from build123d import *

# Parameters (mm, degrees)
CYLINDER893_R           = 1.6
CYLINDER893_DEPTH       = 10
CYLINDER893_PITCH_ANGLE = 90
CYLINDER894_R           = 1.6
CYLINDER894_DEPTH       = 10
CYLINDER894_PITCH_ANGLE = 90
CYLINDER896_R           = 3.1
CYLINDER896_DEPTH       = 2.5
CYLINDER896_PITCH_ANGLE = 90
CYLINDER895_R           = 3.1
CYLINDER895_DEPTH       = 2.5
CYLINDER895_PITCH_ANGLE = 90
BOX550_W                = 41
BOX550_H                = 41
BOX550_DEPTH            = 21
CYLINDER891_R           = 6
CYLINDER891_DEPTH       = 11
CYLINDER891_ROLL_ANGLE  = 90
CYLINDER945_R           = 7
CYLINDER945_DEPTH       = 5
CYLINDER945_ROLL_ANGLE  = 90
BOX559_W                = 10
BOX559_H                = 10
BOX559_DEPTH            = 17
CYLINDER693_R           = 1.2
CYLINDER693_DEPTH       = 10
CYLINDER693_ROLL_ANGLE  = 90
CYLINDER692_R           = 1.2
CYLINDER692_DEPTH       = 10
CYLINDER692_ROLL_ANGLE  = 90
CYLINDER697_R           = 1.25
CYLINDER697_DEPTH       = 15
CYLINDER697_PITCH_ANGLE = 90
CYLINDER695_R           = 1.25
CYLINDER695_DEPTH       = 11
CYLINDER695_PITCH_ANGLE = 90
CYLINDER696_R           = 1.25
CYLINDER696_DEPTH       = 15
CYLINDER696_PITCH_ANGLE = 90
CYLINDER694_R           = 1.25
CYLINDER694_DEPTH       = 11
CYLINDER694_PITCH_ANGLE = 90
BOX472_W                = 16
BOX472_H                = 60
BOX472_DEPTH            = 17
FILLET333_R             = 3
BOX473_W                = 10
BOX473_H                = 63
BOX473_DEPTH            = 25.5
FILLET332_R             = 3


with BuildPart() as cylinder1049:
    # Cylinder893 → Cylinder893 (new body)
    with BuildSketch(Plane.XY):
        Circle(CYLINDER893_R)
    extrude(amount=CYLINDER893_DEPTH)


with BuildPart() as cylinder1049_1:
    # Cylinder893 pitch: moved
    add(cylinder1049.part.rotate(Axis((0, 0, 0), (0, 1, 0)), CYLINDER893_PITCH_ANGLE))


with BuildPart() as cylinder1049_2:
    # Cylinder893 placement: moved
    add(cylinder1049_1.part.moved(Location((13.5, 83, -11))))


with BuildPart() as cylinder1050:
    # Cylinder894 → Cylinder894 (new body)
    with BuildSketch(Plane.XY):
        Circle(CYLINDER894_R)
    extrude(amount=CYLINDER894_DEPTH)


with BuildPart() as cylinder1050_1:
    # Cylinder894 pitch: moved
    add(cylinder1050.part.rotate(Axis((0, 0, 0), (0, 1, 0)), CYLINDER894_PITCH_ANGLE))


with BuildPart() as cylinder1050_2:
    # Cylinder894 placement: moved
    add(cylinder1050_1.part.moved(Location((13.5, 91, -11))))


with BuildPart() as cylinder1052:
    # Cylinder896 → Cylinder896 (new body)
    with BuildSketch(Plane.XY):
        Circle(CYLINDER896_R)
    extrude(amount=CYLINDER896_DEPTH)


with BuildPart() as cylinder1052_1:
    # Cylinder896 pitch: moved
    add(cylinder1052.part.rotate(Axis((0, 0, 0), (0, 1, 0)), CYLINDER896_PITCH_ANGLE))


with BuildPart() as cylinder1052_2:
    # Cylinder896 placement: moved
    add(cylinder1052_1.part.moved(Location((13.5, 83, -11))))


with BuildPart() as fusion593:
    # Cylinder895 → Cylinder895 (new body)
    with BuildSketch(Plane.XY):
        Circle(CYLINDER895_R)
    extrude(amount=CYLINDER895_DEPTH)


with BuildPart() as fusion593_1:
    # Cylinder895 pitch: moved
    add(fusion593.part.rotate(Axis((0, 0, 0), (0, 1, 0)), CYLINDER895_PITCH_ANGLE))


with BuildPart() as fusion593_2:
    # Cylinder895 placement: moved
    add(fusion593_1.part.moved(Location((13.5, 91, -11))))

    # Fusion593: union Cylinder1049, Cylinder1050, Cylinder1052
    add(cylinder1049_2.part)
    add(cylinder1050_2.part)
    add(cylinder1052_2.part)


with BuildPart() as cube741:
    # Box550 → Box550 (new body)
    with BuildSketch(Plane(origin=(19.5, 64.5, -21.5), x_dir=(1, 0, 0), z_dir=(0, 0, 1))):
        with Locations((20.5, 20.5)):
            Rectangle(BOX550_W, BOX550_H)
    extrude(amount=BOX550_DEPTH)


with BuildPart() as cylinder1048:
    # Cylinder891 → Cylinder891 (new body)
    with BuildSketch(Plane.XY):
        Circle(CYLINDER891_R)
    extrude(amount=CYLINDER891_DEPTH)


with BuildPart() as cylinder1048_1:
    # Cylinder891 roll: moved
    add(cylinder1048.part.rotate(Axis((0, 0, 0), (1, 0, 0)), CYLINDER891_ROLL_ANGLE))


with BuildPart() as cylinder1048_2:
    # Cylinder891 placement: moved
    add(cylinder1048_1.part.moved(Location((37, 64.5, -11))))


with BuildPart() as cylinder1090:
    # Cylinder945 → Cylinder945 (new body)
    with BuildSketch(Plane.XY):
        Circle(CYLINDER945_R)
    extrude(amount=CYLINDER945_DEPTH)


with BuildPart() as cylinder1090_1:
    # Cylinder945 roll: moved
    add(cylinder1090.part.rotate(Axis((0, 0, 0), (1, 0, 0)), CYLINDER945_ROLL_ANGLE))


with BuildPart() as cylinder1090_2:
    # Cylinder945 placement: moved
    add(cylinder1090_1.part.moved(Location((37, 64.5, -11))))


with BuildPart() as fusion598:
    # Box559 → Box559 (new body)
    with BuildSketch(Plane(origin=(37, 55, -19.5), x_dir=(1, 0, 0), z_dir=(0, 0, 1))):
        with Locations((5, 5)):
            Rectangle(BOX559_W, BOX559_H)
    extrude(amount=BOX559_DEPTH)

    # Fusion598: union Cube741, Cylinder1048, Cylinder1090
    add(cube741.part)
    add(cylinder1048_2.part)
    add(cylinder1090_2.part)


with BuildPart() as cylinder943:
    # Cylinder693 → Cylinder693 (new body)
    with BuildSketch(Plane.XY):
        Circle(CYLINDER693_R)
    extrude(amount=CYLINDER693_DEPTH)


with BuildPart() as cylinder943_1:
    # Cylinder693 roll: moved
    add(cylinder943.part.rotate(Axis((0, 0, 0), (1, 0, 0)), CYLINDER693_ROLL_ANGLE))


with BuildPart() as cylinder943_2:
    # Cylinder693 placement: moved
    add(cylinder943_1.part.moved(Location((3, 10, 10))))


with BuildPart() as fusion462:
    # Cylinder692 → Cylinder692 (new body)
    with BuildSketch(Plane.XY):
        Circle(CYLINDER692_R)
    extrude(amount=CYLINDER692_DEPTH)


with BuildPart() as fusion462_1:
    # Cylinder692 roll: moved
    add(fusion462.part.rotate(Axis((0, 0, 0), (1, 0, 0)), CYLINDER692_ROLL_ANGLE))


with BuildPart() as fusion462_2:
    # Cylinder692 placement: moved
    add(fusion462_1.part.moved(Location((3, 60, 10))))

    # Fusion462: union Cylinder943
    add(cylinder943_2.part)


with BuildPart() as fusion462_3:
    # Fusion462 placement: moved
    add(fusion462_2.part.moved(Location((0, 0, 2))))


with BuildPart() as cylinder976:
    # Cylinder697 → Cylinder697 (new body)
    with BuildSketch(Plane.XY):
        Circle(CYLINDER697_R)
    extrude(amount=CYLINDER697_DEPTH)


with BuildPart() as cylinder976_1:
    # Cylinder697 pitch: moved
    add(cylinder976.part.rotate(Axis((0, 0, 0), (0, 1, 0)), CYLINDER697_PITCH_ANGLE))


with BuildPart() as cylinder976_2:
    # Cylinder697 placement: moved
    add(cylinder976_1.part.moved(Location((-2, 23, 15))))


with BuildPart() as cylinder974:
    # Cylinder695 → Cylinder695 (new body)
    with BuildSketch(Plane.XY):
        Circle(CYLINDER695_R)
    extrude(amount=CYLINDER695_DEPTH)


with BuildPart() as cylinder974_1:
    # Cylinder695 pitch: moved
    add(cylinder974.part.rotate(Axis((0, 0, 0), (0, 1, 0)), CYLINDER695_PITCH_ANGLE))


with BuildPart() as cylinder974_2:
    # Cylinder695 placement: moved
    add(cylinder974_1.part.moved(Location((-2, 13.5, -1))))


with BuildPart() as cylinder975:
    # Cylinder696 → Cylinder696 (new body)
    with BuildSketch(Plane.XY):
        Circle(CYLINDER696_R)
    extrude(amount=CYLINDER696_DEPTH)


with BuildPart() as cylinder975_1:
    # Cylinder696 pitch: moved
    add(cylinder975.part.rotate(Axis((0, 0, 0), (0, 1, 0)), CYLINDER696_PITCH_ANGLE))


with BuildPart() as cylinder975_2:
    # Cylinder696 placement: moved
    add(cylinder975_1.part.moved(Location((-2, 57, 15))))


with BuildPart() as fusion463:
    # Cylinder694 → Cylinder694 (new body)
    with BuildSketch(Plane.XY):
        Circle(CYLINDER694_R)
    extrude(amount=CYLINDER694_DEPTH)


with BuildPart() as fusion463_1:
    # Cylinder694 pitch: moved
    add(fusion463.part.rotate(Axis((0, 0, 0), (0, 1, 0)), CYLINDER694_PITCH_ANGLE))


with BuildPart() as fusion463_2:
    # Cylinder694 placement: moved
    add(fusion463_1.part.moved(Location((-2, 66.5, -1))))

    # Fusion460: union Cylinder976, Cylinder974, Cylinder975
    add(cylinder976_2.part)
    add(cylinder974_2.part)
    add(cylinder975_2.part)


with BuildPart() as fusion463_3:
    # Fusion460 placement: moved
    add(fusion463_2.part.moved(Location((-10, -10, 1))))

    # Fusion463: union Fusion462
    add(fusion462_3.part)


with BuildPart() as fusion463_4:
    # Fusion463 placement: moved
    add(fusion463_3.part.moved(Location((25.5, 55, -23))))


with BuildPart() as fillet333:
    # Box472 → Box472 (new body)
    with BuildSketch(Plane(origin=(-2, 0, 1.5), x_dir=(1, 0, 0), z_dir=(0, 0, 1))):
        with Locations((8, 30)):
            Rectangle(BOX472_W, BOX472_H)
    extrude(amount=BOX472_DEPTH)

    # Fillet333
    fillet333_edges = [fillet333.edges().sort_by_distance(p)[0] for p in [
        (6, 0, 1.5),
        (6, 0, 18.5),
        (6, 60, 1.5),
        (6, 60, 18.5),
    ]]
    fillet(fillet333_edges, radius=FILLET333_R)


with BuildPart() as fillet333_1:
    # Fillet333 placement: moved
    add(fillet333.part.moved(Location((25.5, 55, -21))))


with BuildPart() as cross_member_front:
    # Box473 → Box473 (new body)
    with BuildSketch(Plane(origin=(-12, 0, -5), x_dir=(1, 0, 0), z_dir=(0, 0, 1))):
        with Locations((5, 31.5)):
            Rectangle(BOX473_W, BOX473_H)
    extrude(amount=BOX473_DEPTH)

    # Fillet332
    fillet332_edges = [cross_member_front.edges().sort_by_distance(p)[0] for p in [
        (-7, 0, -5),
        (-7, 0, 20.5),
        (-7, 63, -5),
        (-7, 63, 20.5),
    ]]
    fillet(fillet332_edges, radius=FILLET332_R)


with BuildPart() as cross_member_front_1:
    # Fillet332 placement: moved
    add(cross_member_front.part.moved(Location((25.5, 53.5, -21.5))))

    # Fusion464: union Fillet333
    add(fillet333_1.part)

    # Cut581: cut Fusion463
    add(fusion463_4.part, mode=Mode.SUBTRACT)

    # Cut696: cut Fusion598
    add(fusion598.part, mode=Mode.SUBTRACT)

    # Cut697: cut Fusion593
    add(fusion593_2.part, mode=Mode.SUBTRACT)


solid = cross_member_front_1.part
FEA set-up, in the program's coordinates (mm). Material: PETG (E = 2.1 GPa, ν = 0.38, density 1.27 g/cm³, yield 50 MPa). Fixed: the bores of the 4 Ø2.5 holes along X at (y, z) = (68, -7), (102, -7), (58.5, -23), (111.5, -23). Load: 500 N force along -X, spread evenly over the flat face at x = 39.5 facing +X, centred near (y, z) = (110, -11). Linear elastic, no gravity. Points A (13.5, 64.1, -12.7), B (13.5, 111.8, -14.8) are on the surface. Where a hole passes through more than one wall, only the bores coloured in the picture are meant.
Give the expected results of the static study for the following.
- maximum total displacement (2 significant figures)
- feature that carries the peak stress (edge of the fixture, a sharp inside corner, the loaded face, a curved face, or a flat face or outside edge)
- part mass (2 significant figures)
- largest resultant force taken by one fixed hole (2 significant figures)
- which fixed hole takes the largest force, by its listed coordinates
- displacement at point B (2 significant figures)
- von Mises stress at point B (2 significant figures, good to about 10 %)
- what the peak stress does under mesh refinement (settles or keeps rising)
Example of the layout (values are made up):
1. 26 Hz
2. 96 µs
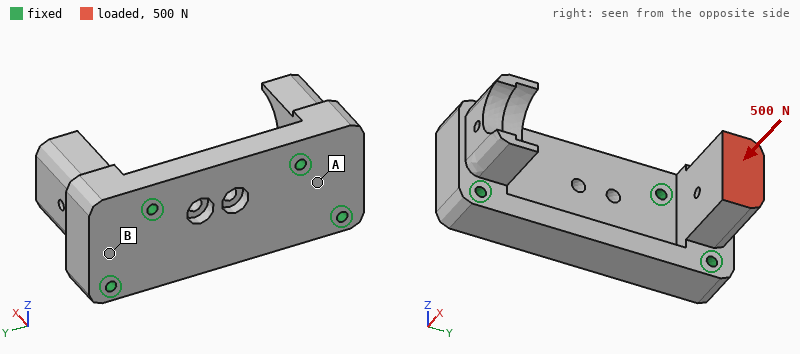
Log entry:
1. 0.21 mm
2. edge of the fixture
3. 21 g
4. 270 N
5. (102, -7)
6. 0.052 mm
7. 3.9 MPa
8. keeps rising
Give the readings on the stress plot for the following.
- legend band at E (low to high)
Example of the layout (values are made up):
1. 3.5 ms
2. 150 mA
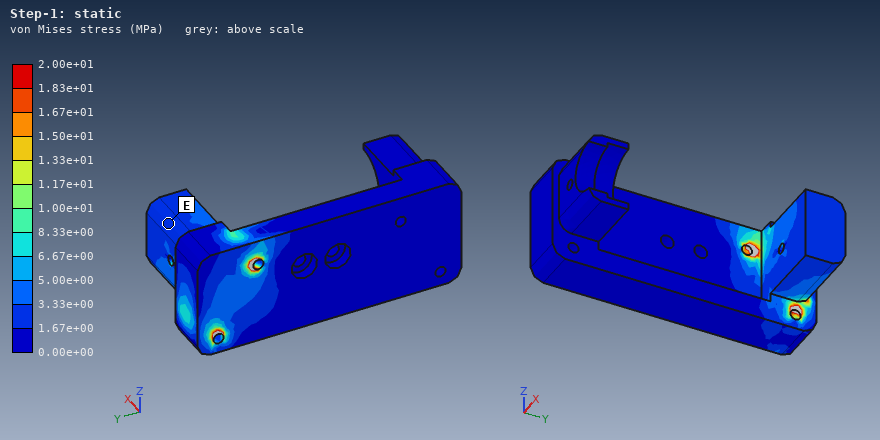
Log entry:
1. 1.67e+00 to 3.33e+00 MPa
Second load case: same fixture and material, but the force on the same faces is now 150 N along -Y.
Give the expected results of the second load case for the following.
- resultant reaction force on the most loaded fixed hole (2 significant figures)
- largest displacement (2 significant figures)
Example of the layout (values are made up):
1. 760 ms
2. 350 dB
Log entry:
1. 120 N
2. 0.43 mm
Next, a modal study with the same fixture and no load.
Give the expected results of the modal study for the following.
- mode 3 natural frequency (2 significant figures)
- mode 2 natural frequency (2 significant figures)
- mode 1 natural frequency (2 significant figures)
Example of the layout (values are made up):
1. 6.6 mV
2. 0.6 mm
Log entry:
1. 4300 Hz
2. 3600 Hz
3. 2500 Hz
